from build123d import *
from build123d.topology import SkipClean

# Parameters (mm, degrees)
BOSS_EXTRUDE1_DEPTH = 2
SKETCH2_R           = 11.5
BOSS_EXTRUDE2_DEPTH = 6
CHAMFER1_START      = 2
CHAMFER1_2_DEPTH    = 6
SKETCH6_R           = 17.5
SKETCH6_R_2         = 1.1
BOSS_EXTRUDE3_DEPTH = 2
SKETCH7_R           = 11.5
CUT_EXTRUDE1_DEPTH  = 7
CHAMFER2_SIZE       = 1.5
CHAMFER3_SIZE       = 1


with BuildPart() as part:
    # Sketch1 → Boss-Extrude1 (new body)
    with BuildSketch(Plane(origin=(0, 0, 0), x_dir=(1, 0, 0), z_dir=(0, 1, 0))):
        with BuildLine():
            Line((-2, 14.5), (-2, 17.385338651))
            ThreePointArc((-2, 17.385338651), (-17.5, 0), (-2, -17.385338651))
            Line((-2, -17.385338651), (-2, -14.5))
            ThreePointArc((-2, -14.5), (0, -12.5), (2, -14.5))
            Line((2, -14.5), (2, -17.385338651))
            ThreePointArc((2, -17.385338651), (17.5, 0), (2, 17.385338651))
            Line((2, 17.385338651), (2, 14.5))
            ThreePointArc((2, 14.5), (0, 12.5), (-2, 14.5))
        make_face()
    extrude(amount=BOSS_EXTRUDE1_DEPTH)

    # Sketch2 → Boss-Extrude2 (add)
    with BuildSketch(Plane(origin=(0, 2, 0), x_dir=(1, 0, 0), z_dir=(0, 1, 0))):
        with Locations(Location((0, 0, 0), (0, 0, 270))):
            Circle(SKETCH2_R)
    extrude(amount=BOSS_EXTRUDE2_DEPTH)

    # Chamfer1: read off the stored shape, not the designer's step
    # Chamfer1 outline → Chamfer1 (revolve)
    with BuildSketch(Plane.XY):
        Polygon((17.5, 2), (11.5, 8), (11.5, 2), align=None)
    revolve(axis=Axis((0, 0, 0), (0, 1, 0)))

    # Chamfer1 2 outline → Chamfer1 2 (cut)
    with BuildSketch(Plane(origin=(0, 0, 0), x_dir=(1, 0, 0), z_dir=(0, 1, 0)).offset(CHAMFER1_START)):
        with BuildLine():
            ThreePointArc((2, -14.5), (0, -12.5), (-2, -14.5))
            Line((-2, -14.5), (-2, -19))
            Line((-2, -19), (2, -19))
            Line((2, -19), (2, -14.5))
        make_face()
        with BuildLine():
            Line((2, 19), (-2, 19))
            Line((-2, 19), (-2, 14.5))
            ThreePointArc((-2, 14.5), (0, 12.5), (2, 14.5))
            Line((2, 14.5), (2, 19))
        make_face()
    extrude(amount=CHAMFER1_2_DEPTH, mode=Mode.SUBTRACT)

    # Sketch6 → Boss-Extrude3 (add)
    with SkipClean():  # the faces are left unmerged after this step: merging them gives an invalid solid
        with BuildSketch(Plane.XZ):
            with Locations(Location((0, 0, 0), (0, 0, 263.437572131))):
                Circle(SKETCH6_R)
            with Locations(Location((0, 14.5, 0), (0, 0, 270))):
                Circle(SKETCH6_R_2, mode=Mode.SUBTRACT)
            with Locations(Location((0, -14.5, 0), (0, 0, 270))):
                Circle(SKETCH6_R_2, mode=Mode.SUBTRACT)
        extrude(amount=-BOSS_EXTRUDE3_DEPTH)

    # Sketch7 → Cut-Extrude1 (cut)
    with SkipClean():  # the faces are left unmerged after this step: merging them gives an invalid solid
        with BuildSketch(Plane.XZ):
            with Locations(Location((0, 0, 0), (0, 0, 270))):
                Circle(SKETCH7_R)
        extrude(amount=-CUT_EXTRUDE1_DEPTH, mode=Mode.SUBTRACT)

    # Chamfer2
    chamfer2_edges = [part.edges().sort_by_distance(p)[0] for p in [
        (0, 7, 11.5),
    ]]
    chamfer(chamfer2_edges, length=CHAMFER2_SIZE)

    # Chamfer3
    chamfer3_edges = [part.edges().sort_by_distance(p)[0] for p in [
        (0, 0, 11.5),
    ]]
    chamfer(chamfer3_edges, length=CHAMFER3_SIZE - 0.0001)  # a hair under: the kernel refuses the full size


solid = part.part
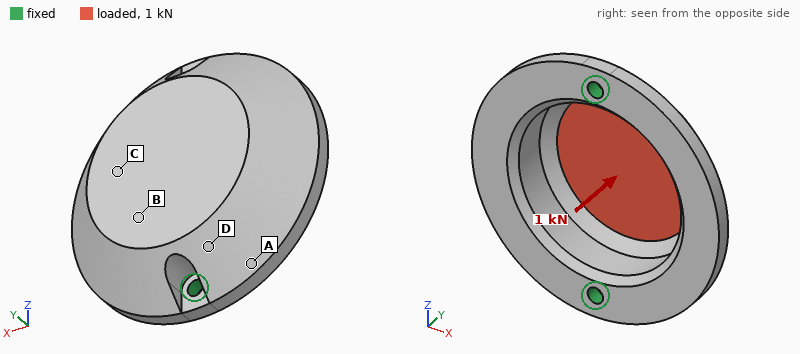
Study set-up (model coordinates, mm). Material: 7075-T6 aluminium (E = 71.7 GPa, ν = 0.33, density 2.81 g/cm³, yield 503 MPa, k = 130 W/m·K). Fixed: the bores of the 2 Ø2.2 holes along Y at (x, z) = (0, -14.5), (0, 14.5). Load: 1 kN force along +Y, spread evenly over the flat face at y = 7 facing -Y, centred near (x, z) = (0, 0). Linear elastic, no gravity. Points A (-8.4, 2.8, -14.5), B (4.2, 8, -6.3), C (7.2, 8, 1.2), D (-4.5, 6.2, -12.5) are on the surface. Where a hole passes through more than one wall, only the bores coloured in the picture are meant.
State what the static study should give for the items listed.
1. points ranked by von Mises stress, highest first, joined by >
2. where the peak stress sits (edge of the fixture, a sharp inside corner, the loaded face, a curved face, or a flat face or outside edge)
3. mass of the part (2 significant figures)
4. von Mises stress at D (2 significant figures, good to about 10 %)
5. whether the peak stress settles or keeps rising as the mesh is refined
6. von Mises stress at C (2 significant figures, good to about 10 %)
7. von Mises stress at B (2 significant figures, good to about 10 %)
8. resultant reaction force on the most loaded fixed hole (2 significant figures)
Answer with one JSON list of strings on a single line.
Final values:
["C > B > D > A", "edge of the fixture", "8.4 g", "38 MPa", "keeps rising", "100 MPa", "78 MPa", "640 N"]
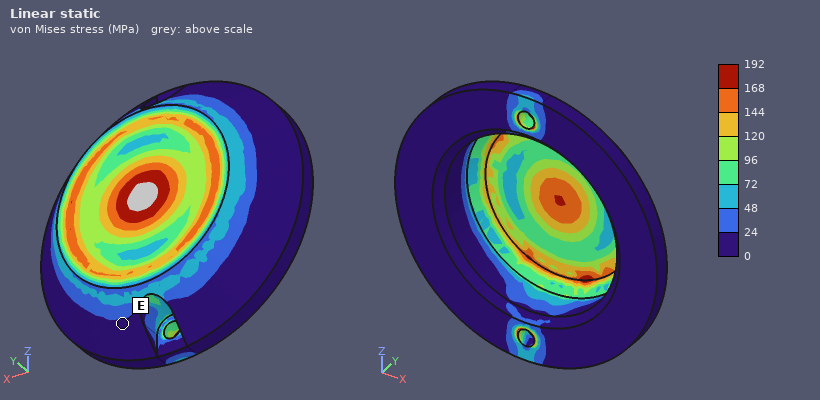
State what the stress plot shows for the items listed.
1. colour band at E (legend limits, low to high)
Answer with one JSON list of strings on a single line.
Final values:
["0 to 24 MPa"]
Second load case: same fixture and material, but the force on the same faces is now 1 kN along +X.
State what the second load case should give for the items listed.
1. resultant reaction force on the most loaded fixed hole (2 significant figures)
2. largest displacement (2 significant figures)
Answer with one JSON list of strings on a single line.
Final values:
["500 N", "0.13 mm"]
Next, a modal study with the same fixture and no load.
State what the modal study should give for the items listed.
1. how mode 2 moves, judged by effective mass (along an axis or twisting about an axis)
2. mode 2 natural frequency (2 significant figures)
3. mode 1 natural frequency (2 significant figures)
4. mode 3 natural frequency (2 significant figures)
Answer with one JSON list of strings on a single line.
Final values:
["along Y", "14 kHz", "4900 Hz", "15 kHz"]
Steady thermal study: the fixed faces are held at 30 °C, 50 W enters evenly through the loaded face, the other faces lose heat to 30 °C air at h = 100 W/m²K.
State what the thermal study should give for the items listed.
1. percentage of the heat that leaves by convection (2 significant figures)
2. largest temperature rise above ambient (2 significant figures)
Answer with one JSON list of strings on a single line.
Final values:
["17 %", "75 K"]
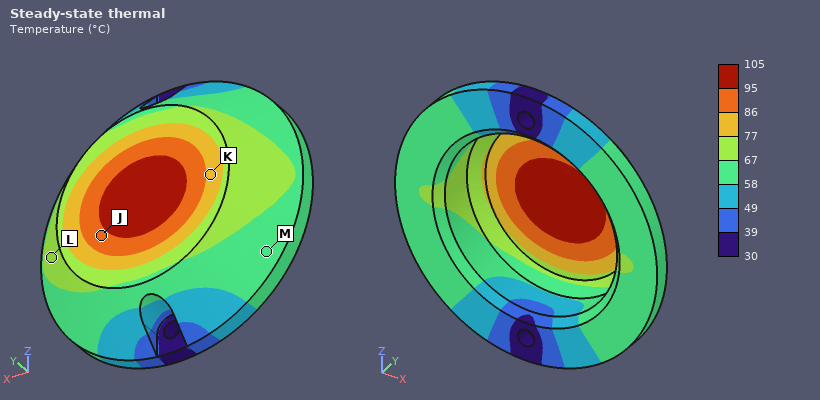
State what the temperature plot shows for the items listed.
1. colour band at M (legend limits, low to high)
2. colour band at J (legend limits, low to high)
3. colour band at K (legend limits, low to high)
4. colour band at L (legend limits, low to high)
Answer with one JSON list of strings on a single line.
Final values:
["58 to 67 °C", "86 to 95 °C", "77 to 86 °C", "67 to 77 °C"]
